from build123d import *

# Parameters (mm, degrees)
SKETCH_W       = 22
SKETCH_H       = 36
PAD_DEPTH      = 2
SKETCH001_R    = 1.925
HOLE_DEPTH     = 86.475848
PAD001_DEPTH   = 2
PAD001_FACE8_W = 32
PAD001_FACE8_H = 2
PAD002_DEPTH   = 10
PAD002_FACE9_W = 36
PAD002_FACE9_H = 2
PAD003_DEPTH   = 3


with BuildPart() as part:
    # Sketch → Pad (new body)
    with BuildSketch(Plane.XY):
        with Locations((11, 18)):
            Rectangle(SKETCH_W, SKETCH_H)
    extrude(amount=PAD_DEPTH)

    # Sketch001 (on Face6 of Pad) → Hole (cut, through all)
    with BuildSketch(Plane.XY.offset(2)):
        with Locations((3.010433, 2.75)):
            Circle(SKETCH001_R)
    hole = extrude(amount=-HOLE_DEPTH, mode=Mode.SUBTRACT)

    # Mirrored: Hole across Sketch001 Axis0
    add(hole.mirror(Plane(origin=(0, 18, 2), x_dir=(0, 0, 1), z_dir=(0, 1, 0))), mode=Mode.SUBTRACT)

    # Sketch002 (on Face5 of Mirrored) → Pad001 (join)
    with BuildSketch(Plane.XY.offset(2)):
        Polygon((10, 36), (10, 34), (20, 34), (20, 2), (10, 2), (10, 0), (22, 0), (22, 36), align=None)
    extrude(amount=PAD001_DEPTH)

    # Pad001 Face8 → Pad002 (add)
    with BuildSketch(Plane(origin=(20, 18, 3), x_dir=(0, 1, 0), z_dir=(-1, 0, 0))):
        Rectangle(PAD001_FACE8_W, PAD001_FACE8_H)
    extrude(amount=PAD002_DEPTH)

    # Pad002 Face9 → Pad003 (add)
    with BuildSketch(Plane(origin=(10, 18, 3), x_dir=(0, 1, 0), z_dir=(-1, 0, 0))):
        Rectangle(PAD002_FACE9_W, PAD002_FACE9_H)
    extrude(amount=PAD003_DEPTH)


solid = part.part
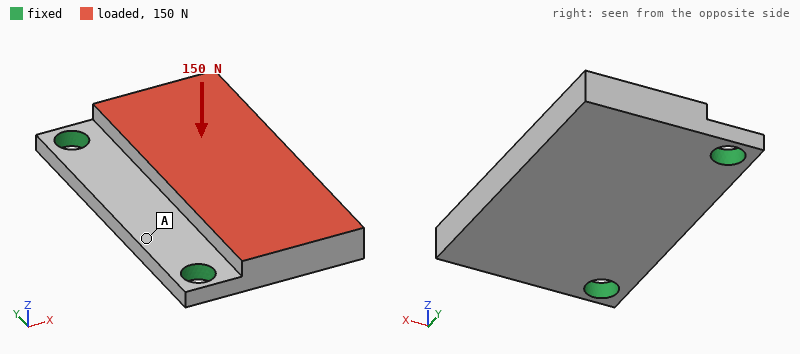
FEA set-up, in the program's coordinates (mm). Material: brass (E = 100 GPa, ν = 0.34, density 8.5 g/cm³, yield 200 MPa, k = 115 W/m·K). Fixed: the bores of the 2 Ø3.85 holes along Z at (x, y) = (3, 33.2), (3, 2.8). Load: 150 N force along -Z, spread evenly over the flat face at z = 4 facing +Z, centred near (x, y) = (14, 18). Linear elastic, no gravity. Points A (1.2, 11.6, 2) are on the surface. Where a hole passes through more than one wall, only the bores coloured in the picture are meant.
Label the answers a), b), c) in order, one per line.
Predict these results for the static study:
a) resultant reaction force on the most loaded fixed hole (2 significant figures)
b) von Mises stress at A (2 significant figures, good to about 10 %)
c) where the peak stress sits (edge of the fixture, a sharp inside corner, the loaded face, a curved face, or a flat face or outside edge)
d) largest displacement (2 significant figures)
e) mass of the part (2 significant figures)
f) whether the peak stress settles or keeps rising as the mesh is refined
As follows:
a) 79 N
b) 19 MPa
c) edge of the fixture
d) 61 µm
e) 22 g
f) keeps rising
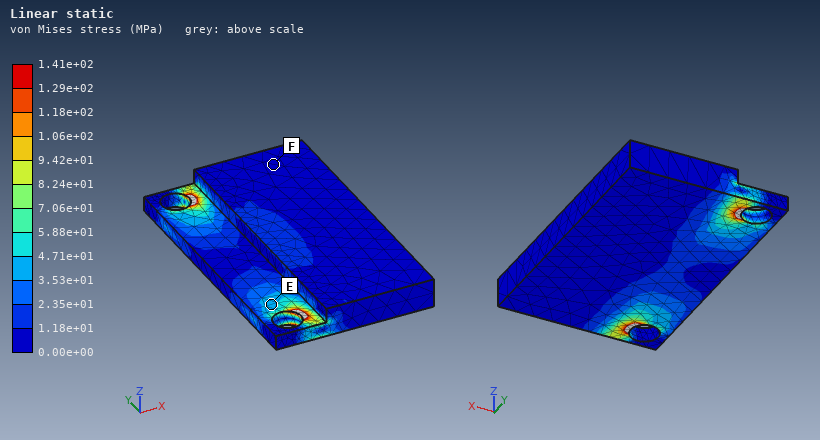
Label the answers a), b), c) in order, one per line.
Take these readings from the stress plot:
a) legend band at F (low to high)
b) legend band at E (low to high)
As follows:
a) 0.00e+00 to 1.18e+01 MPa
b) 3.53e+01 to 4.71e+01 MPa
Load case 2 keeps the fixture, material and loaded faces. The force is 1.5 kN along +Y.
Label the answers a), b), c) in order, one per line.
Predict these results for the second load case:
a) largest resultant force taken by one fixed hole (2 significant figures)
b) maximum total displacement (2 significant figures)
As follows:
a) 920 N
b) 18 µm
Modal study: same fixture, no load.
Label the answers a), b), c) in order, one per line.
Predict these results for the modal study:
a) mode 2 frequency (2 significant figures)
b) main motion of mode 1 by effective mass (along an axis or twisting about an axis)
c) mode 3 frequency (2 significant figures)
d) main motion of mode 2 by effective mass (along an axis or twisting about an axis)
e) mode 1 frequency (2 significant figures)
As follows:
a) 7000 Hz
b) along Z
c) 10 kHz
d) twisting about X
e) 2300 Hz
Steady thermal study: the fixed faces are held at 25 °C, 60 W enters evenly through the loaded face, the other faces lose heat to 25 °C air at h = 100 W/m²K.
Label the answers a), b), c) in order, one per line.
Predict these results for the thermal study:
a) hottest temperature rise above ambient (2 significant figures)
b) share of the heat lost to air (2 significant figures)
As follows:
a) 78 K
b) 13 %
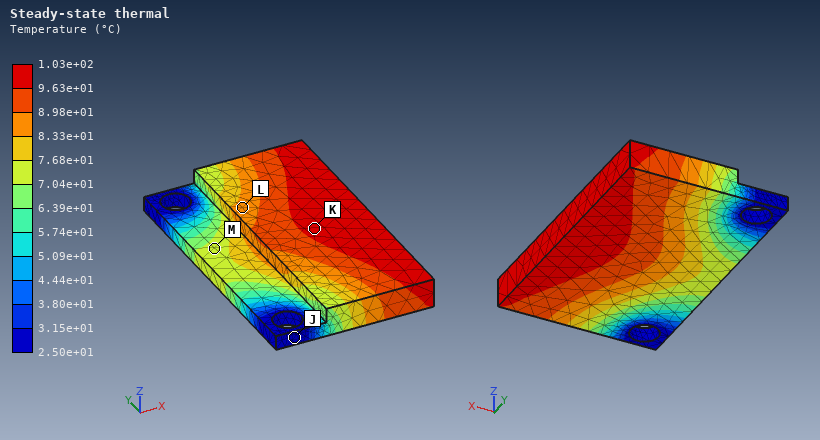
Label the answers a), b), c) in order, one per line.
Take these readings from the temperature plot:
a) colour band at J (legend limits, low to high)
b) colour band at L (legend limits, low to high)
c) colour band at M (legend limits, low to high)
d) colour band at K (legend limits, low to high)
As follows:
a) 2.50e+01 to 3.15e+01 °C
b) 8.33e+01 to 8.98e+01 °C
c) 7.04e+01 to 7.68e+01 °C
d) 9.63e+01 to 1.03e+02 °C
